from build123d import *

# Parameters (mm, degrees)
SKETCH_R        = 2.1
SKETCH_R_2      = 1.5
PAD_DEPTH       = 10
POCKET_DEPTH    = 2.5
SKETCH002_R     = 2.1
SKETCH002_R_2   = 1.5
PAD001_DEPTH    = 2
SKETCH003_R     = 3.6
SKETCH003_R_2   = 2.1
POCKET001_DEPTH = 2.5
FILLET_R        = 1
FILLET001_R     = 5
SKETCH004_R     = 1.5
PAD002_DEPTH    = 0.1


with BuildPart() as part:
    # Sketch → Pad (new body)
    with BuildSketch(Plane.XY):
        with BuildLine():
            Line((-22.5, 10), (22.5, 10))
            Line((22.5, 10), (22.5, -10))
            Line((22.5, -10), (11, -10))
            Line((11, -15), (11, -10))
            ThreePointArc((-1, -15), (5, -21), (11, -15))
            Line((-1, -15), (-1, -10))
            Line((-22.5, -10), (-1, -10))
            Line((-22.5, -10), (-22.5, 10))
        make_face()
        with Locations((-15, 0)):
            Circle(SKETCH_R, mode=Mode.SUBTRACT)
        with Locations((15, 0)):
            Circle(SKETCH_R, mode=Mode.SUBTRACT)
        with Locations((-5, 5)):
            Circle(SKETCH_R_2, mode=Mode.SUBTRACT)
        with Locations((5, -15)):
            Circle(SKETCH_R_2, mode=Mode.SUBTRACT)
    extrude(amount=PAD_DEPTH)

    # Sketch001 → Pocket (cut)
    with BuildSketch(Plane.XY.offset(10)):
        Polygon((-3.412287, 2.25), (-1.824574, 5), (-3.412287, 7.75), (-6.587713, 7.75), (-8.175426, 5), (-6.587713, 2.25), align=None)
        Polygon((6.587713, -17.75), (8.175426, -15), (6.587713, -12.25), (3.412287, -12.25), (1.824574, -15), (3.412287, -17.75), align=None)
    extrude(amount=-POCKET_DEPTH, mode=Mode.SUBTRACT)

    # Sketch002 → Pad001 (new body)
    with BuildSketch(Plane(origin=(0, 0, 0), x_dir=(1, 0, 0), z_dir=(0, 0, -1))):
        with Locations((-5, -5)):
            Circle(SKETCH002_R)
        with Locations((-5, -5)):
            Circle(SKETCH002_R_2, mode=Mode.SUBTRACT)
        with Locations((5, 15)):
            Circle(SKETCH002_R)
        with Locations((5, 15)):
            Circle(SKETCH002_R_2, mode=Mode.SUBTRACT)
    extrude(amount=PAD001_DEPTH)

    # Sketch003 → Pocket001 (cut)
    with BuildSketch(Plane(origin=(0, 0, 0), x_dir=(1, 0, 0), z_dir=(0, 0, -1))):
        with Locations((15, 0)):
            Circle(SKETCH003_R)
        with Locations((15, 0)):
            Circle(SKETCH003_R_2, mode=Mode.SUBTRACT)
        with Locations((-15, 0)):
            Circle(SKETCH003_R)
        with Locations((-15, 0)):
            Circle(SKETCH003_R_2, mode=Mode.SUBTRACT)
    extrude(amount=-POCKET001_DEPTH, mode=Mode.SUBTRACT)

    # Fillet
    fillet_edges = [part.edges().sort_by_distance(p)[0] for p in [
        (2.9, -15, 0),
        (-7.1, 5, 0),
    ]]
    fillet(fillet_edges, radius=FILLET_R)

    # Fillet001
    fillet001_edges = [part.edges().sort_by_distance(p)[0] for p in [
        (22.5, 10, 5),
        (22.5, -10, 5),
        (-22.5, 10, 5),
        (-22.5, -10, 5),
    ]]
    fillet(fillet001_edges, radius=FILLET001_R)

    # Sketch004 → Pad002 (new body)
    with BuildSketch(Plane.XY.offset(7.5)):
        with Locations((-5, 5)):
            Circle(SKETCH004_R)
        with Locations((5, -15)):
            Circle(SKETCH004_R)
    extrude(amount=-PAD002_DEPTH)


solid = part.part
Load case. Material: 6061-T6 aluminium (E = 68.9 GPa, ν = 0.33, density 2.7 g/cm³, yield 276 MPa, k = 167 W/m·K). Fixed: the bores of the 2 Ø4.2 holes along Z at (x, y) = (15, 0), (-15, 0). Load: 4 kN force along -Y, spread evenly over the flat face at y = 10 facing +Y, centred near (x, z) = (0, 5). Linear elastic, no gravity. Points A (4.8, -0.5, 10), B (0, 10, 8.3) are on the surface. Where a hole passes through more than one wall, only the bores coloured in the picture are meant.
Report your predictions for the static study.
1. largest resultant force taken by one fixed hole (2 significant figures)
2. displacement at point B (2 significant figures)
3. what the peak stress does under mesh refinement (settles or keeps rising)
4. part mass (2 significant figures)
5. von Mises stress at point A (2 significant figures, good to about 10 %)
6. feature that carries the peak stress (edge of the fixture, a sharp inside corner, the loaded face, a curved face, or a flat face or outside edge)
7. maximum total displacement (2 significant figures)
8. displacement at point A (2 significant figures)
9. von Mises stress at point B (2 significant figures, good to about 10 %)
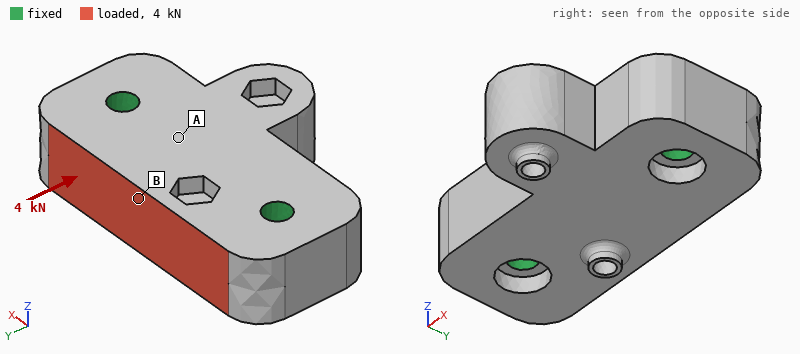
2.0 kN
5.7 µm
keeps rising
25 g
8.1 MPa
edge of the fixture
7.4 µm
3.4 µm
16 MPa
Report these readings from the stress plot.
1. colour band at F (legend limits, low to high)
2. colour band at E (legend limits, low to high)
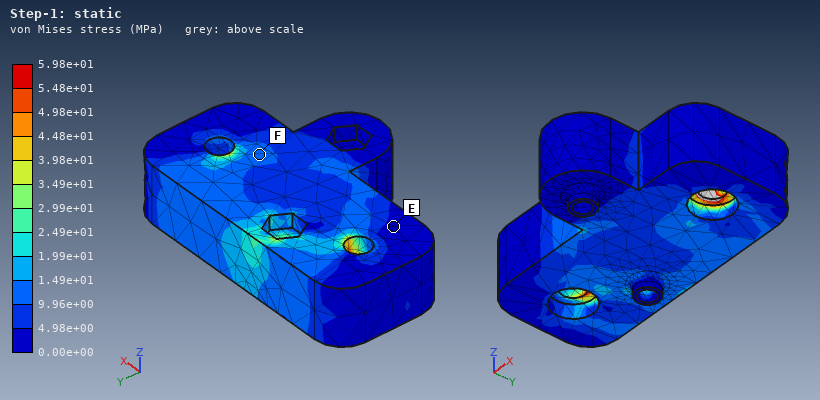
9.96e+00 to 1.49e+01 MPa
0.00e+00 to 4.98e+00 MPa
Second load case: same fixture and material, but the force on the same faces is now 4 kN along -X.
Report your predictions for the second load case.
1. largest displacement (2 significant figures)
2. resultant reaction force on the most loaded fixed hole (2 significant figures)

6.4 µm
2.4 kN
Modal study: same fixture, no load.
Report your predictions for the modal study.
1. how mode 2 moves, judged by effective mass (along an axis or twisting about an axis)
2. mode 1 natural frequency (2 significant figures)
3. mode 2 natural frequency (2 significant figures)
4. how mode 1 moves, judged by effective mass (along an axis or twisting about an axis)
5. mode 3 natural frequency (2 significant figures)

along Z
16 kHz
28 kHz
along Z
30 kHz
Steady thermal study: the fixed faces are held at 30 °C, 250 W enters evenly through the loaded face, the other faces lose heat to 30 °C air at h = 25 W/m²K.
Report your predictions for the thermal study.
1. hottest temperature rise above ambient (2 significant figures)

68 K
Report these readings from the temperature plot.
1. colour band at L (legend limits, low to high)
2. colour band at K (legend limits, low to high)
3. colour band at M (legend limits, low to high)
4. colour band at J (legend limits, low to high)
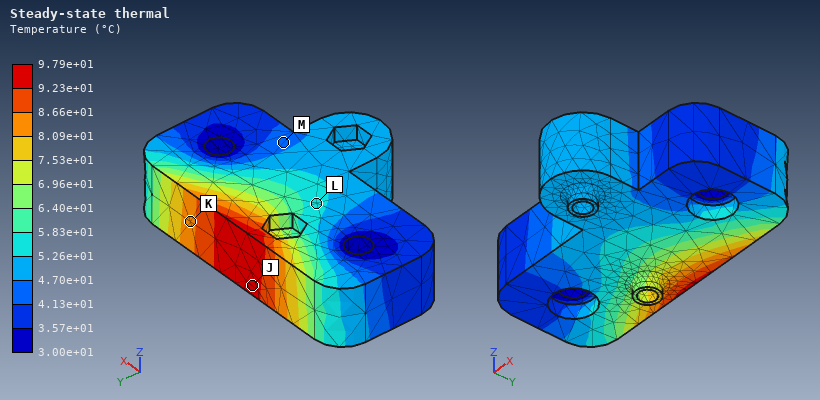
5.26e+01 to 5.83e+01 °C
8.09e+01 to 8.66e+01 °C
4.13e+01 to 4.70e+01 °C
9.23e+01 to 9.79e+01 °C
